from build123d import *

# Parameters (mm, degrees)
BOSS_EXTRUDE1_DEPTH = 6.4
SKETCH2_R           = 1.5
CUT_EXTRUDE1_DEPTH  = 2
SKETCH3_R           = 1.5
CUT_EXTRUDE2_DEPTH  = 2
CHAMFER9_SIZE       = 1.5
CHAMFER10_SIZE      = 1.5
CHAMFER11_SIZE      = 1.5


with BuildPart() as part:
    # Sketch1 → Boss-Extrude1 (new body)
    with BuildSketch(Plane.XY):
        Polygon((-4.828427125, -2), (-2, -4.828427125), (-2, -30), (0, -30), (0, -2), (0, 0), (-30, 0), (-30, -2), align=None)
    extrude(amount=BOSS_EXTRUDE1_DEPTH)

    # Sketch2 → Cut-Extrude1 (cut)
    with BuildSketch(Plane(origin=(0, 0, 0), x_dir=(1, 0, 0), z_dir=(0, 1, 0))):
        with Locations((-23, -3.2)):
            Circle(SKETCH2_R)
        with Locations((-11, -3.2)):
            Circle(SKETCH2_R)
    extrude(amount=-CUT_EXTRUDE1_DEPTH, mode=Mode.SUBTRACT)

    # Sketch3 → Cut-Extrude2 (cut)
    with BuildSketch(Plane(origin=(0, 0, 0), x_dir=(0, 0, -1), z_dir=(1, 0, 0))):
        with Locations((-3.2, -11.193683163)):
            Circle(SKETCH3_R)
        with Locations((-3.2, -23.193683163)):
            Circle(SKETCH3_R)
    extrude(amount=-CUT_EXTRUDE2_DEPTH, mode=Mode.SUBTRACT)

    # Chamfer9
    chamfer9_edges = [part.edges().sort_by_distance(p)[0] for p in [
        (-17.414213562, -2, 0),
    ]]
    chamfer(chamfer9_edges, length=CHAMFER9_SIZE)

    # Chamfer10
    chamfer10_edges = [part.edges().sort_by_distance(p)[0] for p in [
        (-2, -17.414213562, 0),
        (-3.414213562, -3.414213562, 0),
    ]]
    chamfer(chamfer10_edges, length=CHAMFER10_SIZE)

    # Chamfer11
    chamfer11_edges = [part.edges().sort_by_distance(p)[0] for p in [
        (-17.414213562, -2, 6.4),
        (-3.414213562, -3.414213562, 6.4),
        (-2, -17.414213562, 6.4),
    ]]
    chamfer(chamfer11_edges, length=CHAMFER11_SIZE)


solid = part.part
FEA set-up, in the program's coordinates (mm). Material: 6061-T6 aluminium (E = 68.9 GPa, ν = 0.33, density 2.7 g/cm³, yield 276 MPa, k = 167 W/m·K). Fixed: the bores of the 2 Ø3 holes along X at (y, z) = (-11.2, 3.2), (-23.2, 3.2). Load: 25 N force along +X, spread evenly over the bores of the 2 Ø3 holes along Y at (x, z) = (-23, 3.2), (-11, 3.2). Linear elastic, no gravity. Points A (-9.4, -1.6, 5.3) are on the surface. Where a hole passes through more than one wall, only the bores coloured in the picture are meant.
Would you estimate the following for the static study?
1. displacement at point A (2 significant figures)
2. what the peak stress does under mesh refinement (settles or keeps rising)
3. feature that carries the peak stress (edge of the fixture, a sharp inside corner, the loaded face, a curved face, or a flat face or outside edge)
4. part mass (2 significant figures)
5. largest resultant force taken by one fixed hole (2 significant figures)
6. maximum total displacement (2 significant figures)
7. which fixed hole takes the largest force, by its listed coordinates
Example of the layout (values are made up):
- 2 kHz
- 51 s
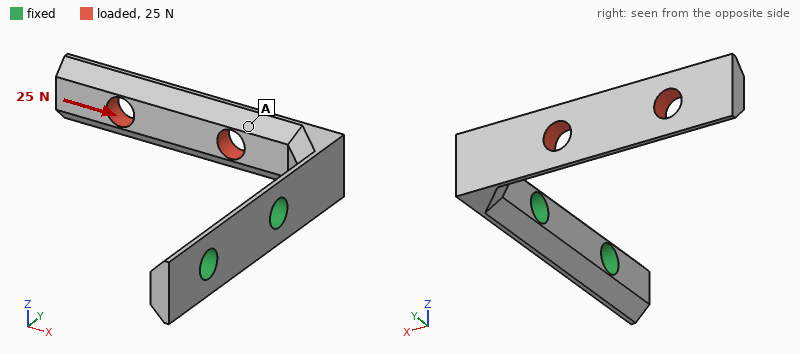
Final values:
- 0.042 mm
- keeps rising
- edge of the fixture
- 1.6 g
- 25 N
- 0.12 mm
- (-11.2, 3.2)
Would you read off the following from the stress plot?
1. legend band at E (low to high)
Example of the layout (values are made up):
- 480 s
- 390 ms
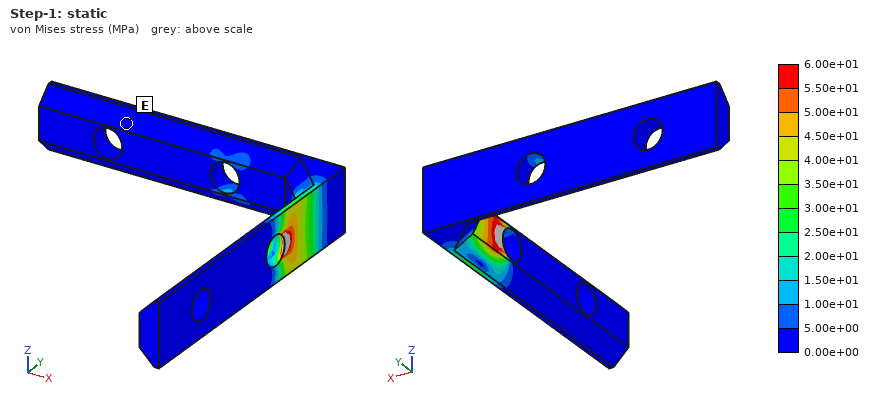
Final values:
- 0.00e+00 to 5.00e+00 MPa
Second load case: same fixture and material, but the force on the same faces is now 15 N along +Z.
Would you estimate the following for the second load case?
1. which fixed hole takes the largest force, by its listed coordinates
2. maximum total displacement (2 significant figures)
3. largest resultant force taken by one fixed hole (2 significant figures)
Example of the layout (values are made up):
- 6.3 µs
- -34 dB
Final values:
- (-11.2, 3.2)
- 0.18 mm
- 17 N
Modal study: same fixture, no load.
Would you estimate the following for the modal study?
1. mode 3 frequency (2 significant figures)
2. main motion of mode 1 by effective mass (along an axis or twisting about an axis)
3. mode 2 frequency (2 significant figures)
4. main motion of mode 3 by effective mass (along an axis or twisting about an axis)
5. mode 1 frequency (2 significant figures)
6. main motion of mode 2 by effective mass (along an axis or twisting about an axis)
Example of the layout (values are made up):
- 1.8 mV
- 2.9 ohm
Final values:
- 5900 Hz
- along Y
- 2200 Hz
- along X
- 1500 Hz
- along Z
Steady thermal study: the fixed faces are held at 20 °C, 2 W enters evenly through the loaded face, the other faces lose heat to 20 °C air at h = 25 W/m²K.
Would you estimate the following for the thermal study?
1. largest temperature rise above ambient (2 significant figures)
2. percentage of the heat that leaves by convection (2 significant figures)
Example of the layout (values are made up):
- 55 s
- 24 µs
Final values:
- 26 K
- 11 %
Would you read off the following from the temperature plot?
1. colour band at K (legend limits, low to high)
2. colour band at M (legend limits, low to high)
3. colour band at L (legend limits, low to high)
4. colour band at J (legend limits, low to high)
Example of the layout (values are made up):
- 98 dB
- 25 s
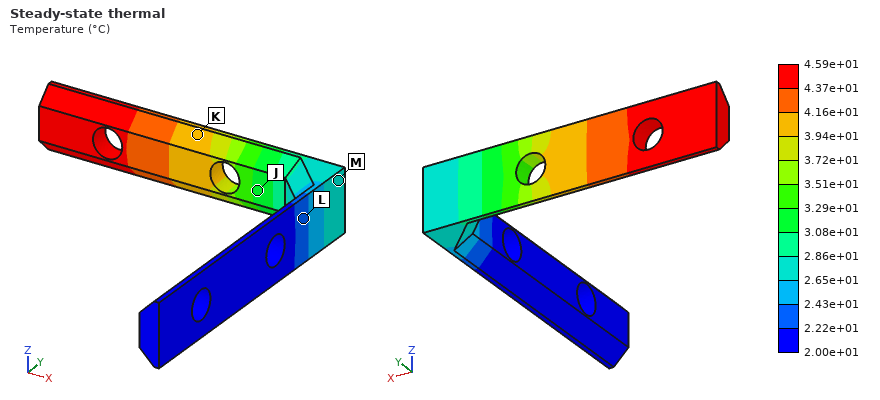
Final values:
- 3.94e+01 to 4.16e+01 °C
- 2.65e+01 to 2.86e+01 °C
- 2.22e+01 to 2.43e+01 °C
- 3.08e+01 to 3.29e+01 °C
